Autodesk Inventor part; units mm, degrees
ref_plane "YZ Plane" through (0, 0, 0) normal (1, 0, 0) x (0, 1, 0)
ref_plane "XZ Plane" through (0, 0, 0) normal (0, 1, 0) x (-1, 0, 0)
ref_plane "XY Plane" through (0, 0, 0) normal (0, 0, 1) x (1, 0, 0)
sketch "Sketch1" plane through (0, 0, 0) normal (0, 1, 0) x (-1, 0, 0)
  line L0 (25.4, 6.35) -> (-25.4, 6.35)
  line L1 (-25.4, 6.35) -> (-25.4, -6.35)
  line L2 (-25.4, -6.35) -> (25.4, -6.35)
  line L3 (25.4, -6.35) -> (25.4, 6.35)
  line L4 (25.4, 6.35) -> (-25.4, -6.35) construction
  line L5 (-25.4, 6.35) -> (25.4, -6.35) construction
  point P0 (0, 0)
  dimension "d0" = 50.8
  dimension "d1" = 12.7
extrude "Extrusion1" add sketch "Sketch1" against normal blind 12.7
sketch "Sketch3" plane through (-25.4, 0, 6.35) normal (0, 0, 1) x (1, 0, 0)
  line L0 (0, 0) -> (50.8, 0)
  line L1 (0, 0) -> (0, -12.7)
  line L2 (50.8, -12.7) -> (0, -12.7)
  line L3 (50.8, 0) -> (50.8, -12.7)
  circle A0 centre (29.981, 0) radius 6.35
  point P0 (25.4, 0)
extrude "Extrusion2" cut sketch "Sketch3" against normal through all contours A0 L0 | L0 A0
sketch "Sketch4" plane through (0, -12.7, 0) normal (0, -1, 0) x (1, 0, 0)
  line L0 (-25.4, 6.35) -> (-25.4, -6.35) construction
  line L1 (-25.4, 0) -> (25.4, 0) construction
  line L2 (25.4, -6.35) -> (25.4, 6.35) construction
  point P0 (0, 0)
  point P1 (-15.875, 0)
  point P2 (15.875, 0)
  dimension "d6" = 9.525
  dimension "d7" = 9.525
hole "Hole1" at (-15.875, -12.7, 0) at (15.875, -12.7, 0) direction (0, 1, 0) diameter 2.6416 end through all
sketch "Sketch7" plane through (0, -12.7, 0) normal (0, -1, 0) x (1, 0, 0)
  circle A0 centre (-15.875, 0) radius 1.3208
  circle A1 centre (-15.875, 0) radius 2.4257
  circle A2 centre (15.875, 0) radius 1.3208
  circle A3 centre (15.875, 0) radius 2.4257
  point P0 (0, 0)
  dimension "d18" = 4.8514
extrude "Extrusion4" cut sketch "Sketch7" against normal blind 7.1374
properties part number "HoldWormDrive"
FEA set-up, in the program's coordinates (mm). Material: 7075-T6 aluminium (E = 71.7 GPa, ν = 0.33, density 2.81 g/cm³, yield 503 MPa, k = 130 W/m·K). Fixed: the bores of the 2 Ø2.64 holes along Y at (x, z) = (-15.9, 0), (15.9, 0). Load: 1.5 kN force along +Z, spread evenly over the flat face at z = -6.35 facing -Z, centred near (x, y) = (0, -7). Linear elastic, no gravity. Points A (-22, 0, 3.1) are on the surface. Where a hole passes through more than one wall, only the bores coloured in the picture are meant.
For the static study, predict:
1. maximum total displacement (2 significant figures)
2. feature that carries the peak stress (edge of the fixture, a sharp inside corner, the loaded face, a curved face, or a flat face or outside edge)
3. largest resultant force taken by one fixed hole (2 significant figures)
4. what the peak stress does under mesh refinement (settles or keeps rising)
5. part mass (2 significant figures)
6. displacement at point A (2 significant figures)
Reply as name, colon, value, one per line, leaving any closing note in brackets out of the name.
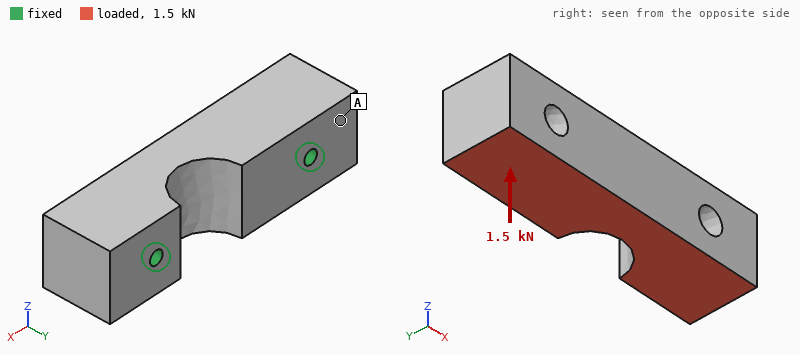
maximum total displacement: 9.5 µm
feature that carries the peak stress: edge of the fixture
largest resultant force taken by one fixed hole: 780 N
what the peak stress does under mesh refinement: keeps rising
part mass: 20 g
displacement at point A: 1.9 µm
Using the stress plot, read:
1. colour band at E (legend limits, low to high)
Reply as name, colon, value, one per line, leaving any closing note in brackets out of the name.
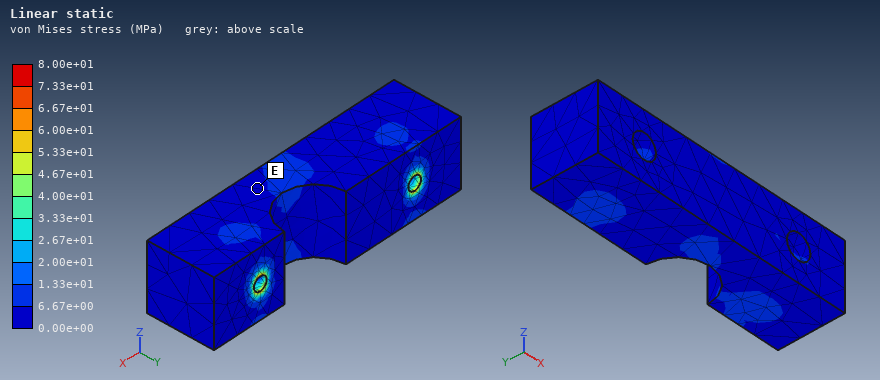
colour band at E: 0.00e+00 to 6.67e+00 MPa
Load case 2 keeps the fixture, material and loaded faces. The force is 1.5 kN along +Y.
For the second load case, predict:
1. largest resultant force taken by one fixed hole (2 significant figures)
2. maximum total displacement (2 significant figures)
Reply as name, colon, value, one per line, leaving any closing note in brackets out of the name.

largest resultant force taken by one fixed hole: 800 N
maximum total displacement: 15 µm
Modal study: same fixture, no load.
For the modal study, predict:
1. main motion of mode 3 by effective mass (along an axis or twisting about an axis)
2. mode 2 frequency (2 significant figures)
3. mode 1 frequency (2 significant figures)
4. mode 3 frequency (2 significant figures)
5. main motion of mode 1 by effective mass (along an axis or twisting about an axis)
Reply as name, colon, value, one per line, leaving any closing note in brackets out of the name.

main motion of mode 3 by effective mass: twisting about Y
mode 2 frequency: 22 kHz
mode 1 frequency: 16 kHz
mode 3 frequency: 24 kHz
main motion of mode 1 by effective mass: along Z
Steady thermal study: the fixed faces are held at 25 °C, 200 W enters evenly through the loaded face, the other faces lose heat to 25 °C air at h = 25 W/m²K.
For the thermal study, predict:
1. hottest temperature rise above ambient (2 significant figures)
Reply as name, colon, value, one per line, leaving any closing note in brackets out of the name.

hottest temperature rise above ambient: 62 K
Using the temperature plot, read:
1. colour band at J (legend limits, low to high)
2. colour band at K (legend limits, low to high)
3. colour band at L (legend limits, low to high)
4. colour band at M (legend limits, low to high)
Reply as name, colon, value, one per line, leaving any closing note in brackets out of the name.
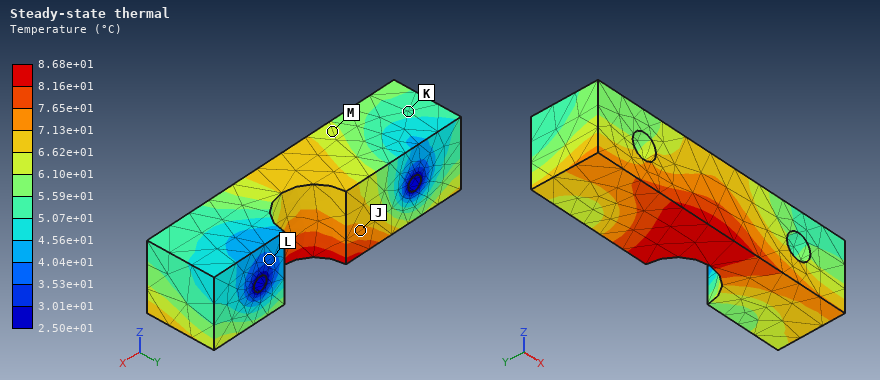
colour band at J: 7.13e+01 to 7.65e+01 °C
colour band at K: 5.07e+01 to 5.59e+01 °C
colour band at L: 3.53e+01 to 4.04e+01 °C
colour band at M: 6.10e+01 to 6.62e+01 °C
